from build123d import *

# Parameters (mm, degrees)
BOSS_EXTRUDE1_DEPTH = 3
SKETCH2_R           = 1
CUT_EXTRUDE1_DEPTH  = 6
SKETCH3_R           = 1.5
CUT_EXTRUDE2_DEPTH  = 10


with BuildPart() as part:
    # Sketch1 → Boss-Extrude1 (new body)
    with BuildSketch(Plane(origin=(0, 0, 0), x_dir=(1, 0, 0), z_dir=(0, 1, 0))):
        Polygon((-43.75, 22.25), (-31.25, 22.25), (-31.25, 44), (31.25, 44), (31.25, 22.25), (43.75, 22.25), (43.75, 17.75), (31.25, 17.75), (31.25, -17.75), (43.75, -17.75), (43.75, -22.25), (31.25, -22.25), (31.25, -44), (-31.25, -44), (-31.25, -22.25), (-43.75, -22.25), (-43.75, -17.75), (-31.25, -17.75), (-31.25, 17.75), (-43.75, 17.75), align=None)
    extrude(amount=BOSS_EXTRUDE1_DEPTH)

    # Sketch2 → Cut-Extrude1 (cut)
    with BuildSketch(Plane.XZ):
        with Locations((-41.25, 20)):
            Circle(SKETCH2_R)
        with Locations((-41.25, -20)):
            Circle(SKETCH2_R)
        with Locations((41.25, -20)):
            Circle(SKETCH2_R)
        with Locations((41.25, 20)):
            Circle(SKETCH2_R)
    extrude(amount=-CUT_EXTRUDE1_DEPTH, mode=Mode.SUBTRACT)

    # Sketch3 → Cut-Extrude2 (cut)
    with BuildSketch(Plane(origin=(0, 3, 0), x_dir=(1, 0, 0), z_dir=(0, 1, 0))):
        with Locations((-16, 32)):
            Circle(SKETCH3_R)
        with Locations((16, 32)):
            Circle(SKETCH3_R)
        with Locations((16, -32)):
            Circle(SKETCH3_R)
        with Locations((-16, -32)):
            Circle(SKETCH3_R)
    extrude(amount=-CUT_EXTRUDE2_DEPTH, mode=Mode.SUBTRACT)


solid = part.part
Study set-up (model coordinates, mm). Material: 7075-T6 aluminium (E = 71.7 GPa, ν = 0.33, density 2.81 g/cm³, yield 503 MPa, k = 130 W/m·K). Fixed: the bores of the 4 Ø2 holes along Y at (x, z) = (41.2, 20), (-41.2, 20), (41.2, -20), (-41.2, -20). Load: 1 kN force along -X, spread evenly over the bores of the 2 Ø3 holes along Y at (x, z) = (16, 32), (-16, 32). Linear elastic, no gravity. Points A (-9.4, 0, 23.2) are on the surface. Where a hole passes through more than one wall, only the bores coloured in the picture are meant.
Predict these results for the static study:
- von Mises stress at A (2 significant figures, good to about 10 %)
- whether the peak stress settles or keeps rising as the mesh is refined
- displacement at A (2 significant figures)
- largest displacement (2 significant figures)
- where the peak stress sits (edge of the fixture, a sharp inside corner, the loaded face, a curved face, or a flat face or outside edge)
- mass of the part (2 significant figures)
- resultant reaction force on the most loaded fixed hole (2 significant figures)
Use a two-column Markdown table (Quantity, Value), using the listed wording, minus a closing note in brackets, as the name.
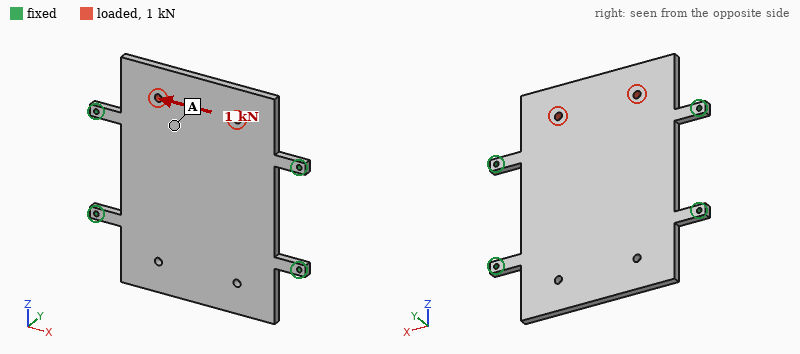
| Quantity | Value |
|---|---|
| von Mises stress at A | 7.1 MPa |
| whether the peak stress settles or keeps rising as the mesh is refined | keeps rising |
| displacement at A | 9.7 µm |
| largest displacement | 18 µm |
| where the peak stress sits | edge of the fixture |
| mass of the part | 48 g |
| resultant reaction force on the most loaded fixed hole | 530 N |
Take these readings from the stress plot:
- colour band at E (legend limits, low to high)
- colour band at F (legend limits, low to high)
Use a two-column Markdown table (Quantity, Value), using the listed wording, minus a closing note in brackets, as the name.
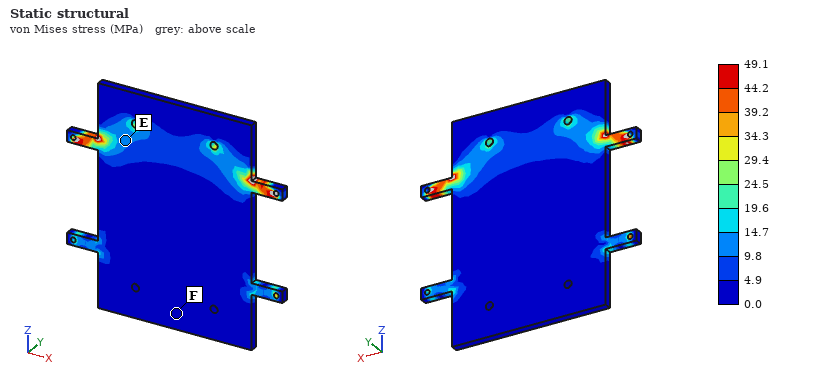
| Quantity | Value |
|---|---|
| colour band at E | 9.8 to 14.7 MPa |
| colour band at F | 0.0 to 4.9 MPa |
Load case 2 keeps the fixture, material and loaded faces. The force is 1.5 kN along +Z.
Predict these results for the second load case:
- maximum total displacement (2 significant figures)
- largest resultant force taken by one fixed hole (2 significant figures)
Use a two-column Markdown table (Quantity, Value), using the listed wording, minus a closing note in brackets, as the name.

| Quantity | Value |
|---|---|
| maximum total displacement | 51 µm |
| largest resultant force taken by one fixed hole | 380 N |
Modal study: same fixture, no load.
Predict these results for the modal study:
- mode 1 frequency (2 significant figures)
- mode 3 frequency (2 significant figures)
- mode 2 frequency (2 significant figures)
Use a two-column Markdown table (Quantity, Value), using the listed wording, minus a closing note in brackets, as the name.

| Quantity | Value |
|---|---|
| mode 1 frequency | 1200 Hz |
| mode 3 frequency | 2500 Hz |
| mode 2 frequency | 1200 Hz |
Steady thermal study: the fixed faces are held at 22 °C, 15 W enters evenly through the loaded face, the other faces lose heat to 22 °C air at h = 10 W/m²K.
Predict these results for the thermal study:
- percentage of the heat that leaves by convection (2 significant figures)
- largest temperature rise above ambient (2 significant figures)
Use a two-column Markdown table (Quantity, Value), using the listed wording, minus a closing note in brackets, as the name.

| Quantity | Value |
|---|---|
| percentage of the heat that leaves by convection | 19 % |
| largest temperature rise above ambient | 39 K |
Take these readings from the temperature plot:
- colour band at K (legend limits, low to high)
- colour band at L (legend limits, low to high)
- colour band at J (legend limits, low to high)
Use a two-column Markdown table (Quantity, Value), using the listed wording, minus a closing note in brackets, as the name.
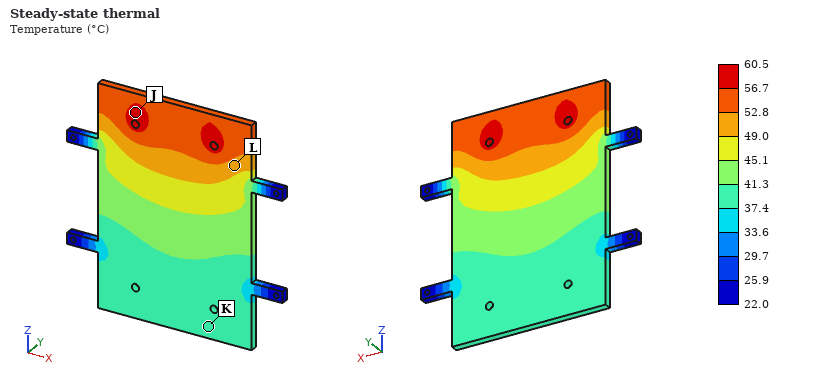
| Quantity | Value |
|---|---|
| colour band at K | 37.4 to 41.3 °C |
| colour band at L | 49.0 to 52.8 °C |
| colour band at J | 56.7 to 60.5 °C |
